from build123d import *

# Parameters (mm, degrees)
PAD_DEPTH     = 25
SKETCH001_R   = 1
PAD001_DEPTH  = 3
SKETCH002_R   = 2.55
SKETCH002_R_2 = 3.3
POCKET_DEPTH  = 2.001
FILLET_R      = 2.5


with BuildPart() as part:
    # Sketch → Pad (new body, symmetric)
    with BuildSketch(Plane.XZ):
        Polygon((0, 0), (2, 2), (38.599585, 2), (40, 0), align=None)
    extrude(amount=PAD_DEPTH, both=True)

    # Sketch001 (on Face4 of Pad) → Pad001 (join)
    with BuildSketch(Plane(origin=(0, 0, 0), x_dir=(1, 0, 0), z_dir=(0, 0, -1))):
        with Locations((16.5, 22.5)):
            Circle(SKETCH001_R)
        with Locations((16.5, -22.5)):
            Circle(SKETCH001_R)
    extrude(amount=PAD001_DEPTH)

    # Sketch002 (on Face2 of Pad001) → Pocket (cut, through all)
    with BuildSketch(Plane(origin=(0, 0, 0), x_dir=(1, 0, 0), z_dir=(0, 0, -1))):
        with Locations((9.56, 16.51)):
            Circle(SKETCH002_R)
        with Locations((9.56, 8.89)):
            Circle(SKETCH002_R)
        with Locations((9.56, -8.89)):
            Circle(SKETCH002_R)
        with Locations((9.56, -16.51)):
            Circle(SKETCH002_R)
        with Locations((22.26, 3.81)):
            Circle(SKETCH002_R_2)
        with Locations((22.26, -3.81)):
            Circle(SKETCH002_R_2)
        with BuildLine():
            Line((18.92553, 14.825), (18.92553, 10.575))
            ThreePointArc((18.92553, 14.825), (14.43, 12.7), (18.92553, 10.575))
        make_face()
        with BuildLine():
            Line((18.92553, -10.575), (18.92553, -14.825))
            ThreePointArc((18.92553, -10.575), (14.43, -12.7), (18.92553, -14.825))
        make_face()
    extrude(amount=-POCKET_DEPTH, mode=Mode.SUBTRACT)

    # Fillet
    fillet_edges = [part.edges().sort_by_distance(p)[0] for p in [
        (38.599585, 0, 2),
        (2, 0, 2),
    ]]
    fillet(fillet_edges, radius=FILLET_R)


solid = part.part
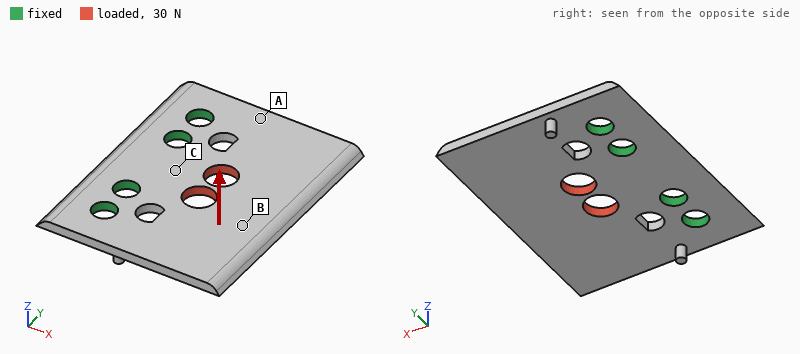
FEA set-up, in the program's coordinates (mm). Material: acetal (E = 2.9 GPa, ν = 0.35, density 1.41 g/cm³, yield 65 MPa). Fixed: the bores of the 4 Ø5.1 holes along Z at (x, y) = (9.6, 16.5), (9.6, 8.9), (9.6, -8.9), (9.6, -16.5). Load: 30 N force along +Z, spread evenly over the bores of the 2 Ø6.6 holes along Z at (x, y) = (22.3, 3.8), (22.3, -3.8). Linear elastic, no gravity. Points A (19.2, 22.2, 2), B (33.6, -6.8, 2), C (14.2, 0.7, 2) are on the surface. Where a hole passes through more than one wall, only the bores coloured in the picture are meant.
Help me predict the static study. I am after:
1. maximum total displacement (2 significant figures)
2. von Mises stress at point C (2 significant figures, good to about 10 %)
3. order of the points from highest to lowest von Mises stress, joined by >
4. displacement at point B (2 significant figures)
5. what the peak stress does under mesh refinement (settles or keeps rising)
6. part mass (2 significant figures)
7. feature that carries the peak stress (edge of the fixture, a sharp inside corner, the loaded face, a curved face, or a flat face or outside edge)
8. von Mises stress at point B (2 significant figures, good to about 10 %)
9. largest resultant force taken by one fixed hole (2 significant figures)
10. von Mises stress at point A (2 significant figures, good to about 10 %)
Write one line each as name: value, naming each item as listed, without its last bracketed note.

maximum total displacement: 0.64 mm
von Mises stress at point C: 8.0 MPa
order of the points from highest to lowest von Mises stress, joined by >: C > A > B
displacement at point B: 0.47 mm
what the peak stress does under mesh refinement: keeps rising
part mass: 4.9 g
feature that carries the peak stress: edge of the fixture
von Mises stress at point B: 2.1 MPa
largest resultant force taken by one fixed hole: 14 N
von Mises stress at point A: 4.7 MPa
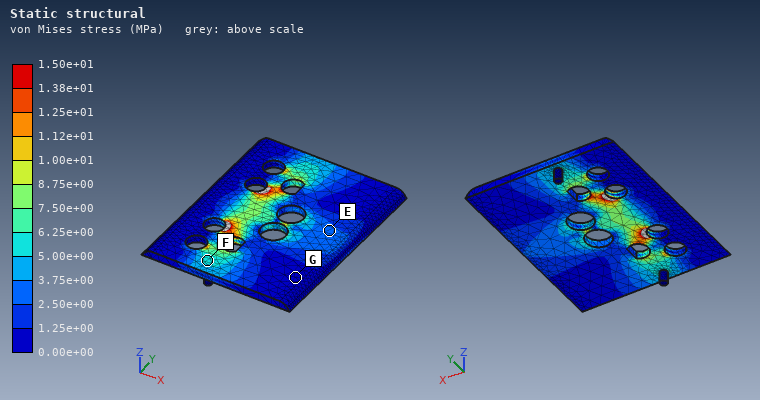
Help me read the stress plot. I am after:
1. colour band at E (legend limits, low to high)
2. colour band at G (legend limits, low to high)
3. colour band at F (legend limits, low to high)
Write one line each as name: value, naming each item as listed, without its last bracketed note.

colour band at E: 2.50e+00 to 3.75e+00 MPa
colour band at G: 0.00e+00 to 1.25e+00 MPa
colour band at F: 5.00e+00 to 6.25e+00 MPa
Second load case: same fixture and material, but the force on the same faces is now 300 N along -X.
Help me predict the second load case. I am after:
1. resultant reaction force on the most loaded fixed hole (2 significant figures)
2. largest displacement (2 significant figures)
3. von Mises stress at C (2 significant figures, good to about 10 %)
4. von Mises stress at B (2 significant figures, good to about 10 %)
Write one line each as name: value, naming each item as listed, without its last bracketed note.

resultant reaction force on the most loaded fixed hole: 120 N
largest displacement: 45 µm
von Mises stress at C: 4.1 MPa
von Mises stress at B: 2.4 MPa
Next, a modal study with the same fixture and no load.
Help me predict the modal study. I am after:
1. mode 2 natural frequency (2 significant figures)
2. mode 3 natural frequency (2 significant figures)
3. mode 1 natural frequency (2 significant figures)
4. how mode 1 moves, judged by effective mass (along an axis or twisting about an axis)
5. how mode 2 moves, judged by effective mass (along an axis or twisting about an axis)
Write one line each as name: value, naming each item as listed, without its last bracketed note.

mode 2 natural frequency: 890 Hz
mode 3 natural frequency: 1800 Hz
mode 1 natural frequency: 530 Hz
how mode 1 moves, judged by effective mass: along Z
how mode 2 moves, judged by effective mass: twisting about X
